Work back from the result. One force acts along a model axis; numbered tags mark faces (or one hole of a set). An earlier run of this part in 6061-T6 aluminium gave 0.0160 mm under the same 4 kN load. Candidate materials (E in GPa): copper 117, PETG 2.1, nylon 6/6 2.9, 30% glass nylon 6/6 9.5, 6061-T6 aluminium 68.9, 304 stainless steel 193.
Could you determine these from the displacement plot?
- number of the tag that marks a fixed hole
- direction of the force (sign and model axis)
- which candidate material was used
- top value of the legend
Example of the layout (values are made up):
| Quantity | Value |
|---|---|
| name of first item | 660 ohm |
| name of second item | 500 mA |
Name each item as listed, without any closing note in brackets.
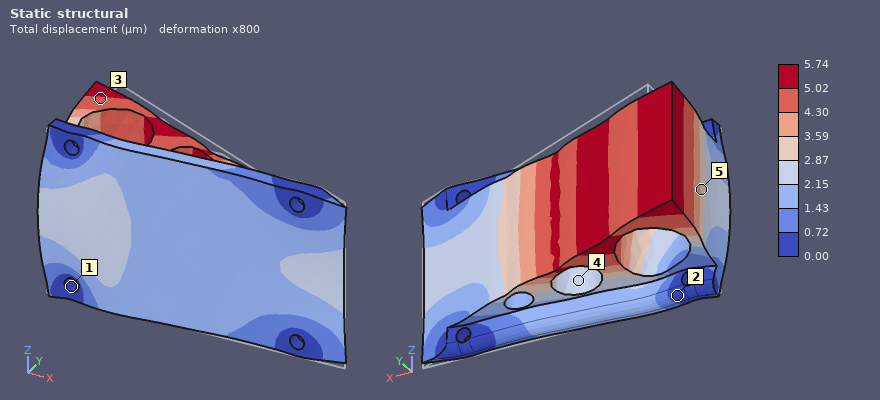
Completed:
| Quantity | Value |
|---|---|
| number of the tag that marks a fixed hole | 1 |
| direction of the force | -X |
| which candidate material was used | 304 stainless steel |
| top value of the legend | 5.74 µm |
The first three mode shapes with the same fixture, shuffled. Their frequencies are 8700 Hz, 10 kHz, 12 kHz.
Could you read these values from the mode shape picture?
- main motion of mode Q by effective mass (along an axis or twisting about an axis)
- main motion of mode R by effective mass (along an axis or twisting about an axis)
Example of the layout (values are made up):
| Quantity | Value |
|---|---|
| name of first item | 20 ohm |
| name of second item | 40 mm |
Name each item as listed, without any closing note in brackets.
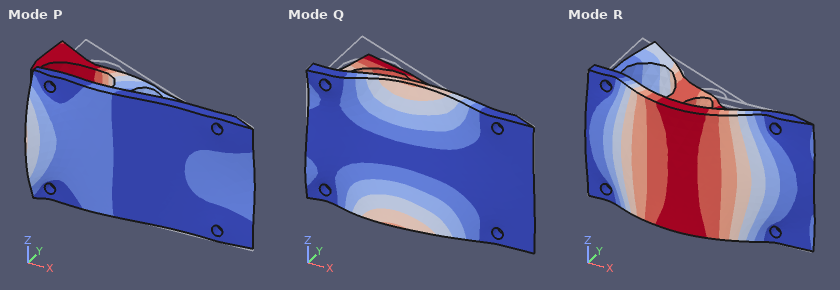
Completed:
| Quantity | Value |
|---|---|
| main motion of mode Q by effective mass | along Z |
| main motion of mode R by effective mass | along Y |
